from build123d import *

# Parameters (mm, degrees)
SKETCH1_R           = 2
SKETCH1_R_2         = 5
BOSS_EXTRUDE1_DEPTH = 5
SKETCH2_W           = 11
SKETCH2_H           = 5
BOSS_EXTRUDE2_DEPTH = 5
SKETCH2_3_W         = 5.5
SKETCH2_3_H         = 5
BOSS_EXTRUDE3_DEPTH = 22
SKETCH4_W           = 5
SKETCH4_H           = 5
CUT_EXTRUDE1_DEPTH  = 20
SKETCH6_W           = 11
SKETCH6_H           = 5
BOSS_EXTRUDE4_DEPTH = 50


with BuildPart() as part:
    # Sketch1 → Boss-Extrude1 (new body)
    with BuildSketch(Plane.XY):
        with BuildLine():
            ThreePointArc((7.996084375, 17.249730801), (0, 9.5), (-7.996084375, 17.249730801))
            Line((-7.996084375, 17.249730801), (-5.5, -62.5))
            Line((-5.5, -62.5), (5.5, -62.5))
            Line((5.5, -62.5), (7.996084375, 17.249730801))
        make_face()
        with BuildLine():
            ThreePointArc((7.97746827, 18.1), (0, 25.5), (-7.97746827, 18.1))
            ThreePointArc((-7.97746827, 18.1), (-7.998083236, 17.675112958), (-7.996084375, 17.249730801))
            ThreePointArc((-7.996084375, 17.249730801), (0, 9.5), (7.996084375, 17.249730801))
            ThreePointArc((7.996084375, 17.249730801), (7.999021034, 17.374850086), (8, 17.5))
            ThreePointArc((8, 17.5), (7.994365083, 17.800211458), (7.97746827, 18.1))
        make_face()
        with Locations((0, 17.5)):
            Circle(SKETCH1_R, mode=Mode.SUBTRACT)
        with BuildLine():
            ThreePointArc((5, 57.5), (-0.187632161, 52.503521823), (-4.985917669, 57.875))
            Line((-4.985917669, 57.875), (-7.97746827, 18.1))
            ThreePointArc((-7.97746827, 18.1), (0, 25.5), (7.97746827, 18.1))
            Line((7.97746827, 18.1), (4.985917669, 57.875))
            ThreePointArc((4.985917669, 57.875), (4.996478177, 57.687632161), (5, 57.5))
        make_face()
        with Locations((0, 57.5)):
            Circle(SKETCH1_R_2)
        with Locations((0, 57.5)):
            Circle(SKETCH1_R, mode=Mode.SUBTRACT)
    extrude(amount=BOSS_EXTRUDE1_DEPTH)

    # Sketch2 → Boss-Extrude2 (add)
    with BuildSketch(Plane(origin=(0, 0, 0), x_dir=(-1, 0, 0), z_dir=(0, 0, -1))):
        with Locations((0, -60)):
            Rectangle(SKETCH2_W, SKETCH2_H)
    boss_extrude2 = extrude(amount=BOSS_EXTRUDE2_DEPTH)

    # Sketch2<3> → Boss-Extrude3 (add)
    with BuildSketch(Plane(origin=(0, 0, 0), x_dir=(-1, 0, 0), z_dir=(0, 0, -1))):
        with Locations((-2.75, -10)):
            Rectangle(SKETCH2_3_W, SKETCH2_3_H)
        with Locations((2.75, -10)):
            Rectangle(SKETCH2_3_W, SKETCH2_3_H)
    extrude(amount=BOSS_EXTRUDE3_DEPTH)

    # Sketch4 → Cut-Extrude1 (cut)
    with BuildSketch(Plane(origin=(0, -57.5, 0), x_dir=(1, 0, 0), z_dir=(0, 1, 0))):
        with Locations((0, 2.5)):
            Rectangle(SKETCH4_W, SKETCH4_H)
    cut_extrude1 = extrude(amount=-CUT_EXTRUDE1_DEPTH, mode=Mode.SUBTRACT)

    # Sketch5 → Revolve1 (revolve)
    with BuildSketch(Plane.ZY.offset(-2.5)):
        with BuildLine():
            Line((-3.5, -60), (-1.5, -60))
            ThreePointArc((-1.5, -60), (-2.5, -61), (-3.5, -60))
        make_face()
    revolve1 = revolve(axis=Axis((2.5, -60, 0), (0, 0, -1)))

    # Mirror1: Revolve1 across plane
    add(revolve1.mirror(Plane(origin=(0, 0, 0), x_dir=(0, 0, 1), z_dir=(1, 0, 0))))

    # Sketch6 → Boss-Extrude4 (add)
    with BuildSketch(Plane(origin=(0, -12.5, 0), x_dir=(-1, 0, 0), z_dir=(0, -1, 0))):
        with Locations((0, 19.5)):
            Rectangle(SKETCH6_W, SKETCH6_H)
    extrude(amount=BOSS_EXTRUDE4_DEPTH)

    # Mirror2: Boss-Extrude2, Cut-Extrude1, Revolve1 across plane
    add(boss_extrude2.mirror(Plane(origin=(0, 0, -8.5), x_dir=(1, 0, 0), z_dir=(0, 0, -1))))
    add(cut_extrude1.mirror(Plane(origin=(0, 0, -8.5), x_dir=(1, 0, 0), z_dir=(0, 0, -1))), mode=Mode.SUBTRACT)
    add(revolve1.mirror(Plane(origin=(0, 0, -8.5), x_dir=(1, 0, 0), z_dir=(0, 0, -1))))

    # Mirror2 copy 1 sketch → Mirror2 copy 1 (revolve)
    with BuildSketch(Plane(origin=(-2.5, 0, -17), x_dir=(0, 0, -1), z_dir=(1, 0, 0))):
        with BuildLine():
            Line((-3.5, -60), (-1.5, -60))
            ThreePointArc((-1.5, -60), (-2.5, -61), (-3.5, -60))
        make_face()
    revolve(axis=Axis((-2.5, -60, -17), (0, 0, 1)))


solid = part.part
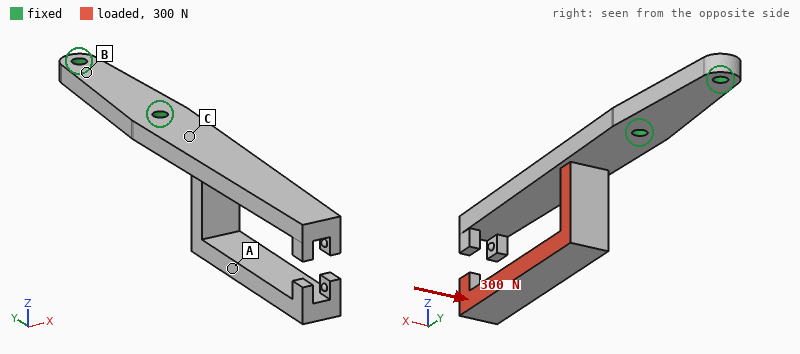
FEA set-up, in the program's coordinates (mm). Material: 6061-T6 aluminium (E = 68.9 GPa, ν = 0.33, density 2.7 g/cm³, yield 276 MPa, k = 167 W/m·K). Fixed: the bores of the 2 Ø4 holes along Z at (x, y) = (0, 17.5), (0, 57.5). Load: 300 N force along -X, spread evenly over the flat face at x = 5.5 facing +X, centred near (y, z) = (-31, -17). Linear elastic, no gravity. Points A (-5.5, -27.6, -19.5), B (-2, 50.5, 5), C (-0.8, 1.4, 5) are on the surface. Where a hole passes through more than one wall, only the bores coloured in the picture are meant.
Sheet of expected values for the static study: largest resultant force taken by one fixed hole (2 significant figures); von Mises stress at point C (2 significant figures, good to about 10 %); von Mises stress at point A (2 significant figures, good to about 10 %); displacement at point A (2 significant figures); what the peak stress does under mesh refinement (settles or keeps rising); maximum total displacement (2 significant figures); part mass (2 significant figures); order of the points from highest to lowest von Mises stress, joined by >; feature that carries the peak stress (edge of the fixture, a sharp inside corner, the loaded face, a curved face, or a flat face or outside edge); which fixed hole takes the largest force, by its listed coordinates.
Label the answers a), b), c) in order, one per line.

a) 510 N
b) 83 MPa
c) 30 MPa
d) 0.63 mm
e) keeps rising
f) 1.3 mm
g) 33 g
h) C > A > B
i) edge of the fixture
j) (0, 17.5)
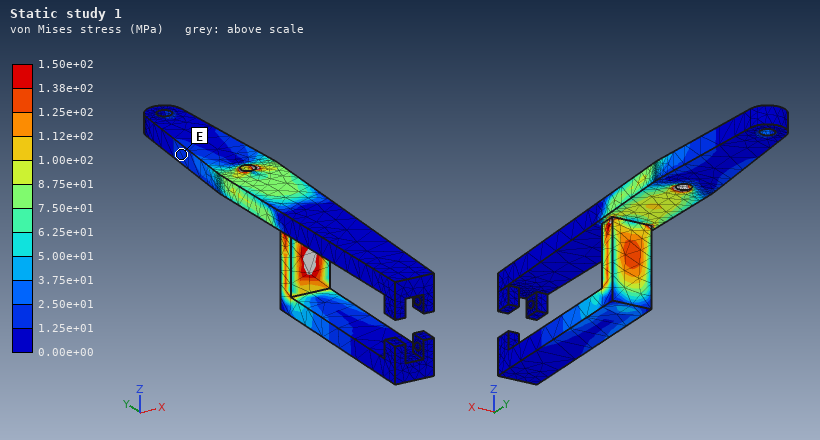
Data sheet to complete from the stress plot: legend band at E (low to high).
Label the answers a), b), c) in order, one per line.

a) 1.25e+01 to 2.50e+01 MPa
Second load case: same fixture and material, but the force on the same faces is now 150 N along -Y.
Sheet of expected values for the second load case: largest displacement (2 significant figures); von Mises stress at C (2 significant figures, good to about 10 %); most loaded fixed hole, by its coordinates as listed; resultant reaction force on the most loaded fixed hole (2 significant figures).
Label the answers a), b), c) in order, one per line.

a) 0.68 mm
b) 43 MPa
c) (0, 17.5)
d) 140 N
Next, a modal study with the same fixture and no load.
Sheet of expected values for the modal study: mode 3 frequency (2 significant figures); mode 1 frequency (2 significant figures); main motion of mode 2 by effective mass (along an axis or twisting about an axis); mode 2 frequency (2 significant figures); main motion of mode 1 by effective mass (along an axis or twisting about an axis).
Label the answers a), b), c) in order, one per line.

a) 1100 Hz
b) 460 Hz
c) along X
d) 870 Hz
e) along Z
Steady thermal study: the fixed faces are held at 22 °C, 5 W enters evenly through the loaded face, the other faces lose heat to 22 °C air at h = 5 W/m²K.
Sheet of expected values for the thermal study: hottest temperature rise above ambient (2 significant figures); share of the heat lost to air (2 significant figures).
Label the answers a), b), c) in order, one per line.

a) 30 K
b) 7.5 %
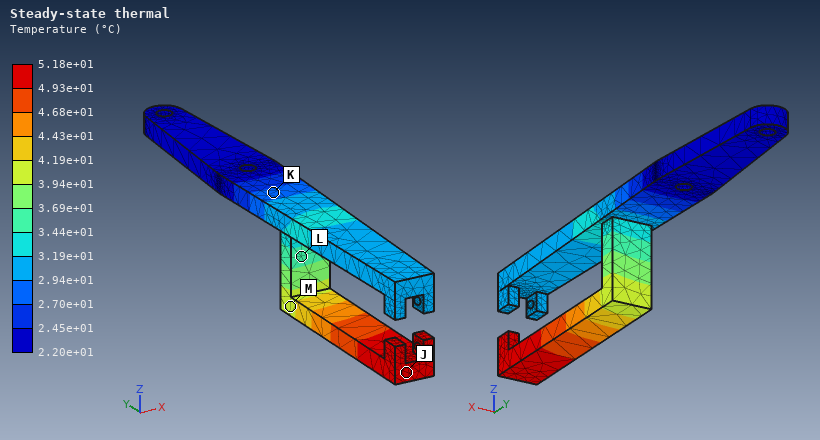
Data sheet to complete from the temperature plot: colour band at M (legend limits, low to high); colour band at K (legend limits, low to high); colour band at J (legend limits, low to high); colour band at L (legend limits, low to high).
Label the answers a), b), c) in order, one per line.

a) 3.94e+01 to 4.19e+01 °C
b) 2.70e+01 to 2.94e+01 °C
c) 4.93e+01 to 5.18e+01 °C
d) 3.44e+01 to 3.69e+01 °C
